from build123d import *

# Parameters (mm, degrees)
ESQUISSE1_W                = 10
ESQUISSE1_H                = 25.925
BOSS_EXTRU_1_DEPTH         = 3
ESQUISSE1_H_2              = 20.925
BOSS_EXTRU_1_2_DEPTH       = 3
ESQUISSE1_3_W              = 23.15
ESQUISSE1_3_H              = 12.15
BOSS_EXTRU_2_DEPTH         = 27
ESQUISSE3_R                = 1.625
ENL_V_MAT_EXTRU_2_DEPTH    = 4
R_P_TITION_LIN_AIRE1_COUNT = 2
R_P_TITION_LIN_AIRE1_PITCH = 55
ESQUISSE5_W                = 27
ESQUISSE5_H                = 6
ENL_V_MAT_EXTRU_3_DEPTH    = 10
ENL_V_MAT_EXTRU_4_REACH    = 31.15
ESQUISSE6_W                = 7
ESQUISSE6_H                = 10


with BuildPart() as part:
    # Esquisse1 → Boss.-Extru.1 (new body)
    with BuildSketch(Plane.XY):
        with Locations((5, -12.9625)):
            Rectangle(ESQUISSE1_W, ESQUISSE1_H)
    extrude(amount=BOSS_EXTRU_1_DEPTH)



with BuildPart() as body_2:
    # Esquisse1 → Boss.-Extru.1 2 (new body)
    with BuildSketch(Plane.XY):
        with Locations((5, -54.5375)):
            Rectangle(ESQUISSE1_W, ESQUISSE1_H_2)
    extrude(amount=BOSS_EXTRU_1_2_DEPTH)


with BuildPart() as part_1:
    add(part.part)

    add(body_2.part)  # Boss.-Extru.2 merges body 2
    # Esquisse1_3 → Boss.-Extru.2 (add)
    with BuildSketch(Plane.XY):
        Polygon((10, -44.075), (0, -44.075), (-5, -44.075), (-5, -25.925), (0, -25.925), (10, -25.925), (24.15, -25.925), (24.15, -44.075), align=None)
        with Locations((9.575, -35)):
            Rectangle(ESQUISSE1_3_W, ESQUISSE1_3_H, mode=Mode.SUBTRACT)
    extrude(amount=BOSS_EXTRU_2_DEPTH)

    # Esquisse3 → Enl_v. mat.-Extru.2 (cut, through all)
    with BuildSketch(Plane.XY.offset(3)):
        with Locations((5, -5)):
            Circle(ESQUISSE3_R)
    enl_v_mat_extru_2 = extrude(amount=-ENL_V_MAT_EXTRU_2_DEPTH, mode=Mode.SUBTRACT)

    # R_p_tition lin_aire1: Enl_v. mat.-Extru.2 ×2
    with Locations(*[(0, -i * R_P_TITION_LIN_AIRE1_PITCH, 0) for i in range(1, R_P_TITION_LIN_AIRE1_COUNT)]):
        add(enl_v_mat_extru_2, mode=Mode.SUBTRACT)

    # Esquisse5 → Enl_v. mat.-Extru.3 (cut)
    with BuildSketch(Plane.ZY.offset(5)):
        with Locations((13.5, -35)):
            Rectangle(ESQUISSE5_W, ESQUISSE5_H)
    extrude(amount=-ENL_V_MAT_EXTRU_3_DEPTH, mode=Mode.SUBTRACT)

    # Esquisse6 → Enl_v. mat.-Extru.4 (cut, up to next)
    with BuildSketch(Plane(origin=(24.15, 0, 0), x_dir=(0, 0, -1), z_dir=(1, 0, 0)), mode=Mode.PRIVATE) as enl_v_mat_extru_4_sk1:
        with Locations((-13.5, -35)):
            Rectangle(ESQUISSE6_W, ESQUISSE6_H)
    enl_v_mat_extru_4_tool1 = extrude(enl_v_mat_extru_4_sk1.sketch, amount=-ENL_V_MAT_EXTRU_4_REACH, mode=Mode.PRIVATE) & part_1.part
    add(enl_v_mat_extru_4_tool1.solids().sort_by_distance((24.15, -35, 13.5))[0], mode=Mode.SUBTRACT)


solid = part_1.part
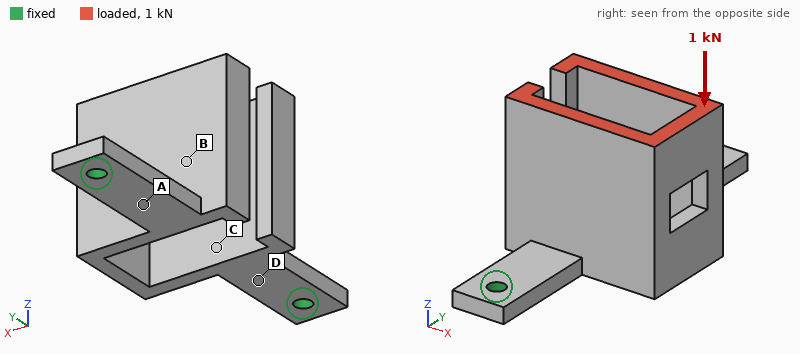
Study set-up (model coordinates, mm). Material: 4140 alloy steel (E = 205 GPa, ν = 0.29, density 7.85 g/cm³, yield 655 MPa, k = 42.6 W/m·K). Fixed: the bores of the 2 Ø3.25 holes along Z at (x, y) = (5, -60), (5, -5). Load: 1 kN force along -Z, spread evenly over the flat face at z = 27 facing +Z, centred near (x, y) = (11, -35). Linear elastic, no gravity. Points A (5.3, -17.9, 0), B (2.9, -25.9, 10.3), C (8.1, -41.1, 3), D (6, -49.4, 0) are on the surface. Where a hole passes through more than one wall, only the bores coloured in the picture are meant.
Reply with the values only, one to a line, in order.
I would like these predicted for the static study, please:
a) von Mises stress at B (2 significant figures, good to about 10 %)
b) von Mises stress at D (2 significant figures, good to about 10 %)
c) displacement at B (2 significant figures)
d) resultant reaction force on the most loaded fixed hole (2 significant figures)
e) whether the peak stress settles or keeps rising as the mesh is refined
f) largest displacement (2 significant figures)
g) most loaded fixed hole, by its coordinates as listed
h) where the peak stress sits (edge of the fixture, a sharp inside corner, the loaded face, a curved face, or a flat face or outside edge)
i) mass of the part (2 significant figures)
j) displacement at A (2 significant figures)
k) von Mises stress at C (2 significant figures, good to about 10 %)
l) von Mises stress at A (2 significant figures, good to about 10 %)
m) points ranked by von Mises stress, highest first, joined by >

57 MPa
210 MPa
0.12 mm
570 N
keeps rising
0.33 mm
(5, -60)
edge of the fixture
58 g
0.062 mm
130 MPa
160 MPa
D > A > C > B
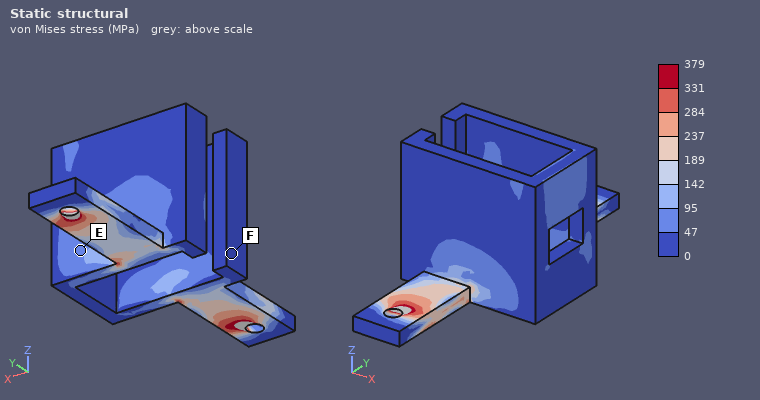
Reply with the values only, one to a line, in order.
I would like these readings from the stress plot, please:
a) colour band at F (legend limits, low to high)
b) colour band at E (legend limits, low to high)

0 to 47 MPa
47 to 95 MPa
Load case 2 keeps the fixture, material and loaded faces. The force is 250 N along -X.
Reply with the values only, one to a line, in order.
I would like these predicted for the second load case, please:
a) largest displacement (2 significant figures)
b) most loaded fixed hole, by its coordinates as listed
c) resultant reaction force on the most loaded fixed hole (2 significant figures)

0.30 mm
(5, -60)
150 N
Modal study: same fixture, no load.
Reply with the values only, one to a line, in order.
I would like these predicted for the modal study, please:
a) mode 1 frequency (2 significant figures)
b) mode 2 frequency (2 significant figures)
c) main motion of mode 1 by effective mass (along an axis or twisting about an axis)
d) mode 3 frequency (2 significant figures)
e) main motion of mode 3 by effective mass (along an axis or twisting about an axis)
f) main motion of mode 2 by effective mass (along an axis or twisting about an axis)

1000 Hz
2200 Hz
along X
2500 Hz
along Y
along Z
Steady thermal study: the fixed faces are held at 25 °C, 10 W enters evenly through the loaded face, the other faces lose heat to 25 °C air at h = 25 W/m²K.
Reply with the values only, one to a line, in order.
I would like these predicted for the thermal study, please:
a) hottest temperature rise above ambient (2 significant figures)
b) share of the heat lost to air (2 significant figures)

61 K
55 %
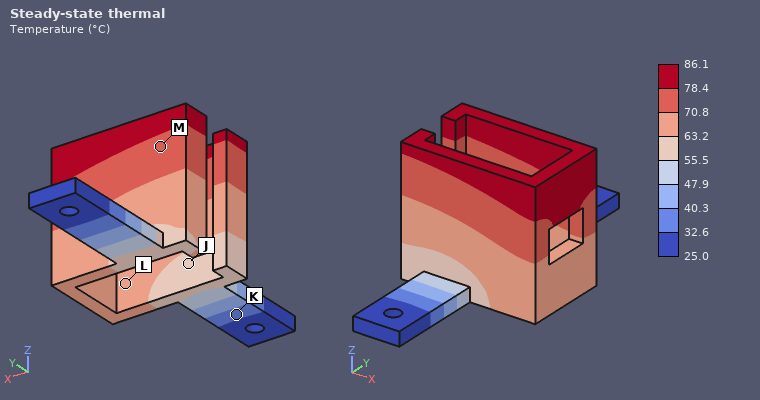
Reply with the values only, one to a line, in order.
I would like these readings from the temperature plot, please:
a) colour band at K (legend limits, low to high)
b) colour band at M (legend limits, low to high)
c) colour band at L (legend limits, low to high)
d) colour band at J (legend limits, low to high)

32.6 to 40.3 °C
70.8 to 78.4 °C
63.2 to 70.8 °C
55.5 to 63.2 °C
